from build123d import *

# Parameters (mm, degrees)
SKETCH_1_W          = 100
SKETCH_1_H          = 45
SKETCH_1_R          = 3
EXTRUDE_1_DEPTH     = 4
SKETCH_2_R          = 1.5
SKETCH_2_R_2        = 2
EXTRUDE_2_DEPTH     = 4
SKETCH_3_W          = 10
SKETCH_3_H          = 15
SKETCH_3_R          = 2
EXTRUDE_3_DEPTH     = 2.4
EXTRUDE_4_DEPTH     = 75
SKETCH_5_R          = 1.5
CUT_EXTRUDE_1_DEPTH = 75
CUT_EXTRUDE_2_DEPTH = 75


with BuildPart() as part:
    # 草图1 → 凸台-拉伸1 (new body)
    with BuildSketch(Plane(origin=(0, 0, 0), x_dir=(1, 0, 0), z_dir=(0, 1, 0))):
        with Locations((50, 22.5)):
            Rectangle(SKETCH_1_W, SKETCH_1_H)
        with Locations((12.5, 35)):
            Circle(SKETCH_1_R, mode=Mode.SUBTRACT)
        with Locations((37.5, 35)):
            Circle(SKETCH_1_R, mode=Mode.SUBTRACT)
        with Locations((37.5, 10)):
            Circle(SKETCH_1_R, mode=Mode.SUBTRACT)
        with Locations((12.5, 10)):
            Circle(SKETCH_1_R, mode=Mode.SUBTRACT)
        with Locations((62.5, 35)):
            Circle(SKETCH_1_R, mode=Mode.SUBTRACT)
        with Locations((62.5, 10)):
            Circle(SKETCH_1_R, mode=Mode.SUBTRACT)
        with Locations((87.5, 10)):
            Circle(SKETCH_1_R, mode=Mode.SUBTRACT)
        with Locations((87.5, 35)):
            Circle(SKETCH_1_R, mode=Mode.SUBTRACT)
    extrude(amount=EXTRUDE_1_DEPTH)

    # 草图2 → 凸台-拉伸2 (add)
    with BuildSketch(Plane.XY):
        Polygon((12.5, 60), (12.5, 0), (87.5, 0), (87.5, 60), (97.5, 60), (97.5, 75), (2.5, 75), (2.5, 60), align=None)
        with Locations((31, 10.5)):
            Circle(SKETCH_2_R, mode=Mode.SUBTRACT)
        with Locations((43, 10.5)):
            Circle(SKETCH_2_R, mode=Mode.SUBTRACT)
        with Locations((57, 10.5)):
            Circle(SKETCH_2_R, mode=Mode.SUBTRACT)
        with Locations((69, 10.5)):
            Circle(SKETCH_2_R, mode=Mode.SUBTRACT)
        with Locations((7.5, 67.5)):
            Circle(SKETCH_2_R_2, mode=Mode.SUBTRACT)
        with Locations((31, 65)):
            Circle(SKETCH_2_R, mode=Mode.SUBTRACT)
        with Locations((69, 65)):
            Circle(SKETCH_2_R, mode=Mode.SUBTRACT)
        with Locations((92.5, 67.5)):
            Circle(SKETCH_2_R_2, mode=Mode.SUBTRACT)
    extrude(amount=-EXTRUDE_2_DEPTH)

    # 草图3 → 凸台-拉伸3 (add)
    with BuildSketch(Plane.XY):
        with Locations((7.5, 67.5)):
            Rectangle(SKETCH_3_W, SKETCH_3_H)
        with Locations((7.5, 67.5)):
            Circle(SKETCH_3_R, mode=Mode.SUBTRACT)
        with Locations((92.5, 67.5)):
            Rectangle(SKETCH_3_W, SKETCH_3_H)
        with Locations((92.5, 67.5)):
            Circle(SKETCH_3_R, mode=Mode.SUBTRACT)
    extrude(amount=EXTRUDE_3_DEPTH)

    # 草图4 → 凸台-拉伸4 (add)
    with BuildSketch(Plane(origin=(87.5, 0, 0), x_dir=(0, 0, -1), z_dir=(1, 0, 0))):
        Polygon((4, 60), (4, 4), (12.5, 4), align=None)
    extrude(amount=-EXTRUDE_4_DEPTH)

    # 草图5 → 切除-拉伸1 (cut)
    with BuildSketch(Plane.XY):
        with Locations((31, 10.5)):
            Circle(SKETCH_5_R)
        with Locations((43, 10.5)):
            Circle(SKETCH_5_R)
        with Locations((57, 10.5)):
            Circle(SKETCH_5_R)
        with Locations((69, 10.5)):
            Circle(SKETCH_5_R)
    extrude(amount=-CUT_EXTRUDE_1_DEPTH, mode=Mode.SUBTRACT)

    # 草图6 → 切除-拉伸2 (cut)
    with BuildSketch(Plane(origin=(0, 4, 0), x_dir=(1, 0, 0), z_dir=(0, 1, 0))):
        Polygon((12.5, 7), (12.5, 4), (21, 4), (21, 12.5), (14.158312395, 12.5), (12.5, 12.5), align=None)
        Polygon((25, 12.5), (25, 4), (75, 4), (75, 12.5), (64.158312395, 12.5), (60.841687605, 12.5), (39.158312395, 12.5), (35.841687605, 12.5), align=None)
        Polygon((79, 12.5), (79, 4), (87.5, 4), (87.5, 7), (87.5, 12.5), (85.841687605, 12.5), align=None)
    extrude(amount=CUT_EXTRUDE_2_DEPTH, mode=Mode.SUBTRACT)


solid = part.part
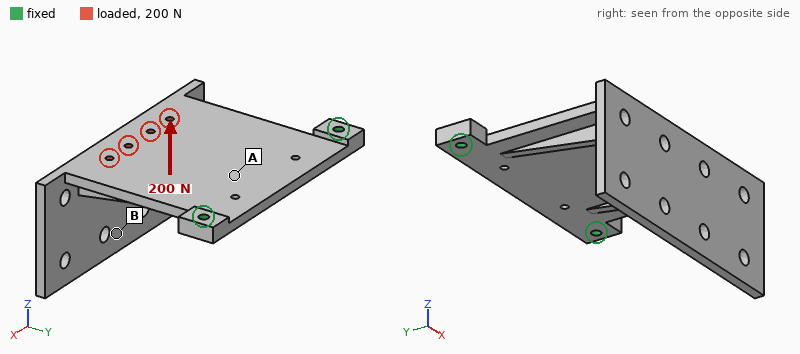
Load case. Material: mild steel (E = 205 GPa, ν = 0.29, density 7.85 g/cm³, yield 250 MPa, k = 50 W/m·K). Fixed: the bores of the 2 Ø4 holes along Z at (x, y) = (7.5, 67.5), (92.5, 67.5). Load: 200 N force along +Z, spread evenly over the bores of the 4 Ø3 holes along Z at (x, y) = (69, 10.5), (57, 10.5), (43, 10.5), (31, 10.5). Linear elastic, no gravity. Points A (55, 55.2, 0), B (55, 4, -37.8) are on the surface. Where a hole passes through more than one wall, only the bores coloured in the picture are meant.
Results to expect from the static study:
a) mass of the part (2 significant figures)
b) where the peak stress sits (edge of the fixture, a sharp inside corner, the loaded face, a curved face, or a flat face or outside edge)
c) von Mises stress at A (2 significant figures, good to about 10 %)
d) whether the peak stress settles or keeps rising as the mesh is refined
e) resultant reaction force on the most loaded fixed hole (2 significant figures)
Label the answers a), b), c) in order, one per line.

a) 330 g
b) a sharp inside corner
c) 23 MPa
d) keeps rising
e) 120 N
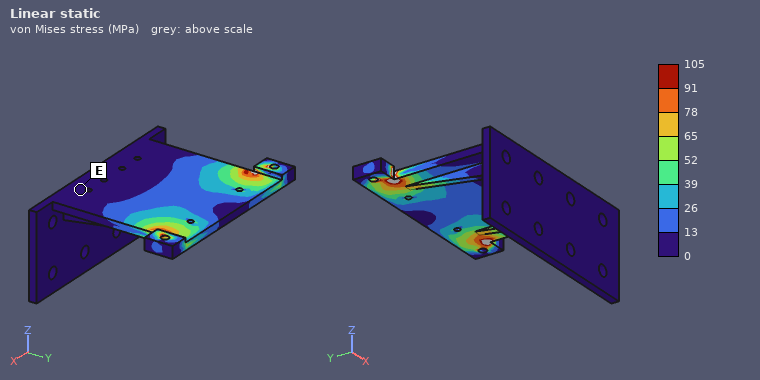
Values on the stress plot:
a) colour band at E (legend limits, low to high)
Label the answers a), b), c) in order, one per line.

a) 0 to 13 MPa
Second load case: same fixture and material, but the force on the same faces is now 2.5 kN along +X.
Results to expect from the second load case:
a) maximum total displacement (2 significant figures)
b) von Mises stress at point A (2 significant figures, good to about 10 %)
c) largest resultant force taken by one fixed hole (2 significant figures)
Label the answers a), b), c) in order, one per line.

a) 25 µm
b) 8.7 MPa
c) 2.2 kN
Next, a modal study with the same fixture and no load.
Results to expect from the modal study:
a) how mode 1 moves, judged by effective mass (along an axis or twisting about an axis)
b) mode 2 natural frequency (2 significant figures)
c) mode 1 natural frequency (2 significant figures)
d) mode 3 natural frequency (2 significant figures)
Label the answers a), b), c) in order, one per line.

a) along Z
b) 680 Hz
c) 280 Hz
d) 1600 Hz
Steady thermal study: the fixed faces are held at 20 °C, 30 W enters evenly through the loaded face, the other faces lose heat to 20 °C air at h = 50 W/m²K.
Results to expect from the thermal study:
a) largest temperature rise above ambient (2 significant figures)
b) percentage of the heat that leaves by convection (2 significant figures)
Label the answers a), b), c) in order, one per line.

a) 51 K
b) 85 %
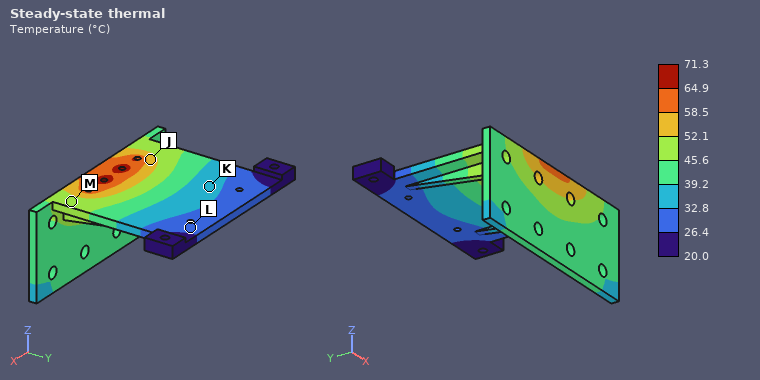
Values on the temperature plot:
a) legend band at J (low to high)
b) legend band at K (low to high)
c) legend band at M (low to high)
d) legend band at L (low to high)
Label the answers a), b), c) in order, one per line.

a) 52.1 to 58.5 °C
b) 32.8 to 39.2 °C
c) 45.6 to 52.1 °C
d) 26.4 to 32.8 °C
